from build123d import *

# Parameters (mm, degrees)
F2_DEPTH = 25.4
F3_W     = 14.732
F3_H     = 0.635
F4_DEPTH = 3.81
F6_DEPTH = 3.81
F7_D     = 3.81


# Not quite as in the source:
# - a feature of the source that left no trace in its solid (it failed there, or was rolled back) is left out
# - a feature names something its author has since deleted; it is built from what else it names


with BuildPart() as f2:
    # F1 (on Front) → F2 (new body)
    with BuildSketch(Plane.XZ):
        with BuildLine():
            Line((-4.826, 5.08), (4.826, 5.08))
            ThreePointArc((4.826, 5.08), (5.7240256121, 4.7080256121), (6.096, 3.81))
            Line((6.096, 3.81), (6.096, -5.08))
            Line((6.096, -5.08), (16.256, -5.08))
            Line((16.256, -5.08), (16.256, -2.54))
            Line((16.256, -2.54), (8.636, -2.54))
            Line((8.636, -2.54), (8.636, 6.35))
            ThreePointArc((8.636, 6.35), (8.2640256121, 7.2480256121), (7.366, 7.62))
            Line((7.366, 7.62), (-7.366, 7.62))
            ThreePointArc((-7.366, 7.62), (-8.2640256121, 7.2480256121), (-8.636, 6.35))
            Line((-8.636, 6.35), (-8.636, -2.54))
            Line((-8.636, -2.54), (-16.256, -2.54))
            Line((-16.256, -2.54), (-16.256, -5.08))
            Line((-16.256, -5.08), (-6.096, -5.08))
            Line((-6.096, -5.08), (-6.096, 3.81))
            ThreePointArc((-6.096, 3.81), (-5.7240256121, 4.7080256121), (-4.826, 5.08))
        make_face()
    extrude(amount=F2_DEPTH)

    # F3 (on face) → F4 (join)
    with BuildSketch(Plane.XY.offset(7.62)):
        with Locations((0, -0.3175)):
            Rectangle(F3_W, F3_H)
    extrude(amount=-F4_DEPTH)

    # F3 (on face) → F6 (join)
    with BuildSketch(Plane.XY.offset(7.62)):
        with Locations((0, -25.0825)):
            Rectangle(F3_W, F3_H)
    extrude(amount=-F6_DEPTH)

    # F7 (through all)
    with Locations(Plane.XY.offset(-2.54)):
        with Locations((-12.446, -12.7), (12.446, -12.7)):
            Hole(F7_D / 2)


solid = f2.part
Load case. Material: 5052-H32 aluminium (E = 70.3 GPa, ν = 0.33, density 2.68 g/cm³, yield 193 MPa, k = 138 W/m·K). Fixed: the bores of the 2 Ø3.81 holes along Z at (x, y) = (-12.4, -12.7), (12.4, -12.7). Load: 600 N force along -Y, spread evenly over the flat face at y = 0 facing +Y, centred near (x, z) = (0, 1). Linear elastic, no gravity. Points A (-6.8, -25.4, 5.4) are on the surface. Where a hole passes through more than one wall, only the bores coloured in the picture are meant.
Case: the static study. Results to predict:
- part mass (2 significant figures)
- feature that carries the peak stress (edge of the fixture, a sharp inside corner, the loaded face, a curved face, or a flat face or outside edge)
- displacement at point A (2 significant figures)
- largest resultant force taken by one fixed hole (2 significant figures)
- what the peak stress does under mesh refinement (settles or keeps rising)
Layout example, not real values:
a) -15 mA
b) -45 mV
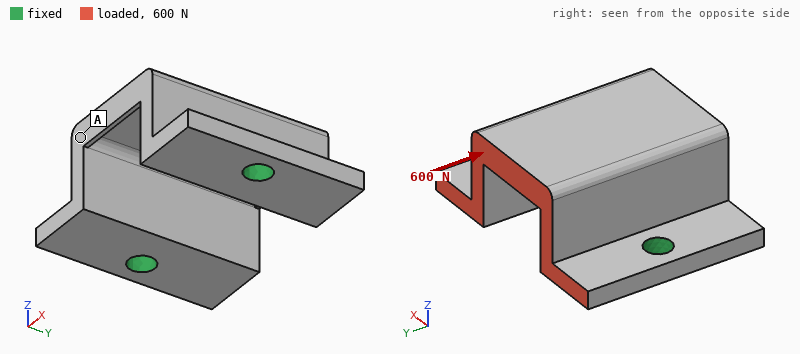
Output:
a) 9.0 g
b) edge of the fixture
c) 34 µm
d) 300 N
e) keeps rising
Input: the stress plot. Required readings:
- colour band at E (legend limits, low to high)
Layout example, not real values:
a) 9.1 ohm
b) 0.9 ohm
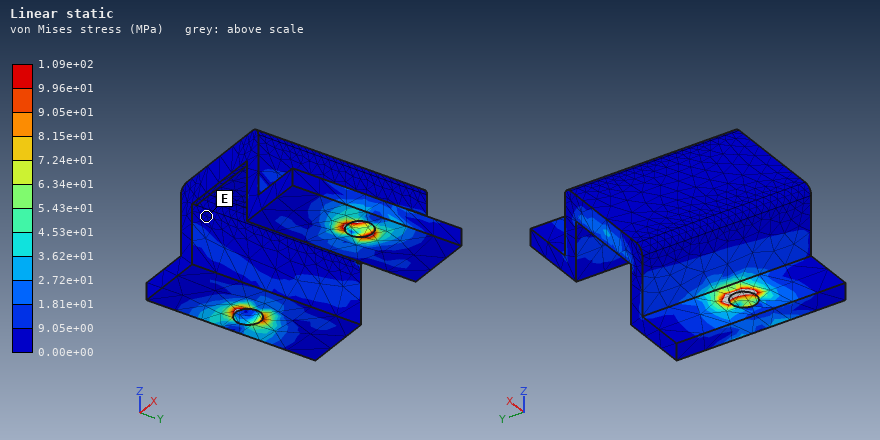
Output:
a) 0.00e+00 to 9.05e+00 MPa
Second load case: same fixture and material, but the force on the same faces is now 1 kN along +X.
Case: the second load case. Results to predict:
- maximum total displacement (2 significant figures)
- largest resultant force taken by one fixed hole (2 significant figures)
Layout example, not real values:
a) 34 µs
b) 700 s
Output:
a) 58 µm
b) 600 N
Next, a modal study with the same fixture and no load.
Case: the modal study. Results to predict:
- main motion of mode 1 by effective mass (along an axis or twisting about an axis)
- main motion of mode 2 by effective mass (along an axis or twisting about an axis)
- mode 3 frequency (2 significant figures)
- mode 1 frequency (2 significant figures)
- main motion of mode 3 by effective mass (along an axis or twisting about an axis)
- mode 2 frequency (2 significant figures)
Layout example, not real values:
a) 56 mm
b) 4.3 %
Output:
a) along Y
b) along X
c) 14 kHz
d) 6800 Hz
e) twisting about Z
f) 13 kHz
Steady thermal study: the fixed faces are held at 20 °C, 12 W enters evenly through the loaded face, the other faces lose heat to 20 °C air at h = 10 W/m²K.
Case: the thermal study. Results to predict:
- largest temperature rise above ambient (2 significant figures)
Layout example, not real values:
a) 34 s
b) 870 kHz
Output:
a) 16 K
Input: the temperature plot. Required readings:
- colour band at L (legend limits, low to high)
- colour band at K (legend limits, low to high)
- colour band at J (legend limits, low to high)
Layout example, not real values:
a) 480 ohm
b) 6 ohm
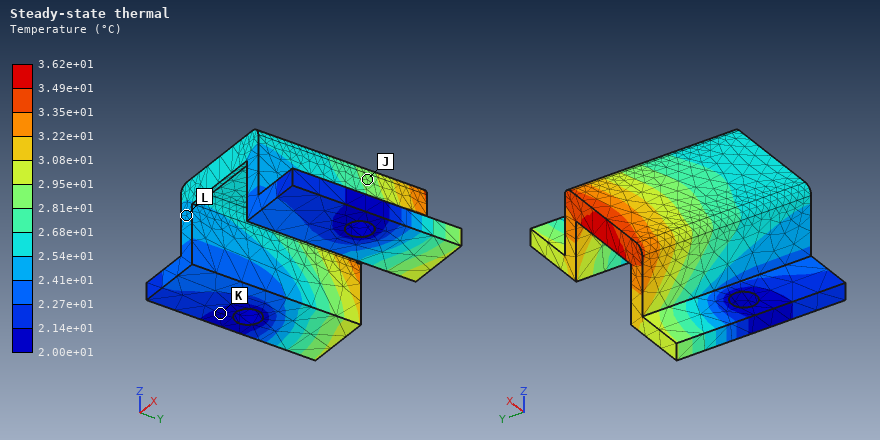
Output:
a) 2.41e+01 to 2.54e+01 °C
b) 2.00e+01 to 2.14e+01 °C
c) 2.81e+01 to 2.95e+01 °C
